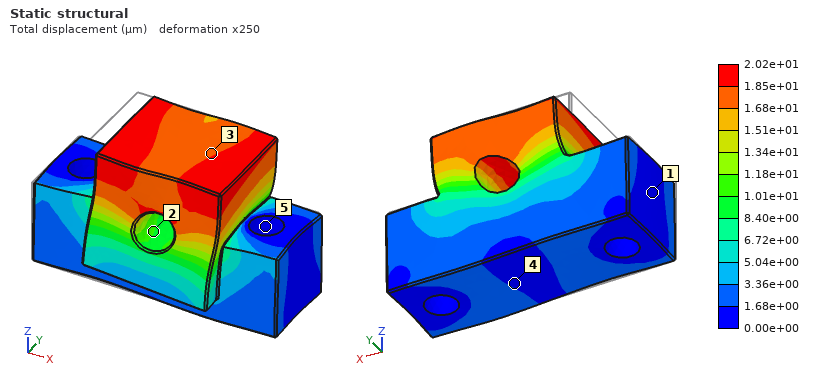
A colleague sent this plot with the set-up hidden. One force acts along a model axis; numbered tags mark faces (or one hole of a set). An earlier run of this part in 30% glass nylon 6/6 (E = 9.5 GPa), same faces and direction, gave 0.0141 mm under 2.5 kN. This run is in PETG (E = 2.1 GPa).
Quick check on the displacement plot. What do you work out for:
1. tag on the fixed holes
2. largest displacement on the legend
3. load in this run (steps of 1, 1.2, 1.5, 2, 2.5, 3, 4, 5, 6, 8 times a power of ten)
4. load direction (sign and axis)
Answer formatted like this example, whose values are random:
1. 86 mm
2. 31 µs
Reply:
1. 5
2. 2.02e+01 µm
3. 800 N
4. +X
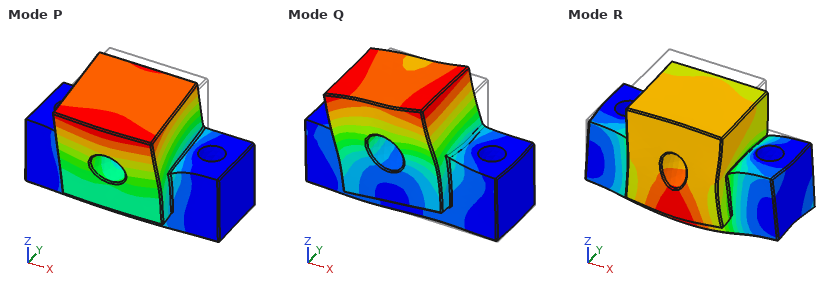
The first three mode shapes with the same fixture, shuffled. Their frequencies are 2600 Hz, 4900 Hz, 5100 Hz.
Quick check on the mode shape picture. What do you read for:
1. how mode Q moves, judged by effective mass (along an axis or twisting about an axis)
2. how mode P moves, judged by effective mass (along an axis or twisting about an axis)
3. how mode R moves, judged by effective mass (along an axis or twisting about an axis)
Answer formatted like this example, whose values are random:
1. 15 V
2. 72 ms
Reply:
1. along X
2. along Y
3. along Z
